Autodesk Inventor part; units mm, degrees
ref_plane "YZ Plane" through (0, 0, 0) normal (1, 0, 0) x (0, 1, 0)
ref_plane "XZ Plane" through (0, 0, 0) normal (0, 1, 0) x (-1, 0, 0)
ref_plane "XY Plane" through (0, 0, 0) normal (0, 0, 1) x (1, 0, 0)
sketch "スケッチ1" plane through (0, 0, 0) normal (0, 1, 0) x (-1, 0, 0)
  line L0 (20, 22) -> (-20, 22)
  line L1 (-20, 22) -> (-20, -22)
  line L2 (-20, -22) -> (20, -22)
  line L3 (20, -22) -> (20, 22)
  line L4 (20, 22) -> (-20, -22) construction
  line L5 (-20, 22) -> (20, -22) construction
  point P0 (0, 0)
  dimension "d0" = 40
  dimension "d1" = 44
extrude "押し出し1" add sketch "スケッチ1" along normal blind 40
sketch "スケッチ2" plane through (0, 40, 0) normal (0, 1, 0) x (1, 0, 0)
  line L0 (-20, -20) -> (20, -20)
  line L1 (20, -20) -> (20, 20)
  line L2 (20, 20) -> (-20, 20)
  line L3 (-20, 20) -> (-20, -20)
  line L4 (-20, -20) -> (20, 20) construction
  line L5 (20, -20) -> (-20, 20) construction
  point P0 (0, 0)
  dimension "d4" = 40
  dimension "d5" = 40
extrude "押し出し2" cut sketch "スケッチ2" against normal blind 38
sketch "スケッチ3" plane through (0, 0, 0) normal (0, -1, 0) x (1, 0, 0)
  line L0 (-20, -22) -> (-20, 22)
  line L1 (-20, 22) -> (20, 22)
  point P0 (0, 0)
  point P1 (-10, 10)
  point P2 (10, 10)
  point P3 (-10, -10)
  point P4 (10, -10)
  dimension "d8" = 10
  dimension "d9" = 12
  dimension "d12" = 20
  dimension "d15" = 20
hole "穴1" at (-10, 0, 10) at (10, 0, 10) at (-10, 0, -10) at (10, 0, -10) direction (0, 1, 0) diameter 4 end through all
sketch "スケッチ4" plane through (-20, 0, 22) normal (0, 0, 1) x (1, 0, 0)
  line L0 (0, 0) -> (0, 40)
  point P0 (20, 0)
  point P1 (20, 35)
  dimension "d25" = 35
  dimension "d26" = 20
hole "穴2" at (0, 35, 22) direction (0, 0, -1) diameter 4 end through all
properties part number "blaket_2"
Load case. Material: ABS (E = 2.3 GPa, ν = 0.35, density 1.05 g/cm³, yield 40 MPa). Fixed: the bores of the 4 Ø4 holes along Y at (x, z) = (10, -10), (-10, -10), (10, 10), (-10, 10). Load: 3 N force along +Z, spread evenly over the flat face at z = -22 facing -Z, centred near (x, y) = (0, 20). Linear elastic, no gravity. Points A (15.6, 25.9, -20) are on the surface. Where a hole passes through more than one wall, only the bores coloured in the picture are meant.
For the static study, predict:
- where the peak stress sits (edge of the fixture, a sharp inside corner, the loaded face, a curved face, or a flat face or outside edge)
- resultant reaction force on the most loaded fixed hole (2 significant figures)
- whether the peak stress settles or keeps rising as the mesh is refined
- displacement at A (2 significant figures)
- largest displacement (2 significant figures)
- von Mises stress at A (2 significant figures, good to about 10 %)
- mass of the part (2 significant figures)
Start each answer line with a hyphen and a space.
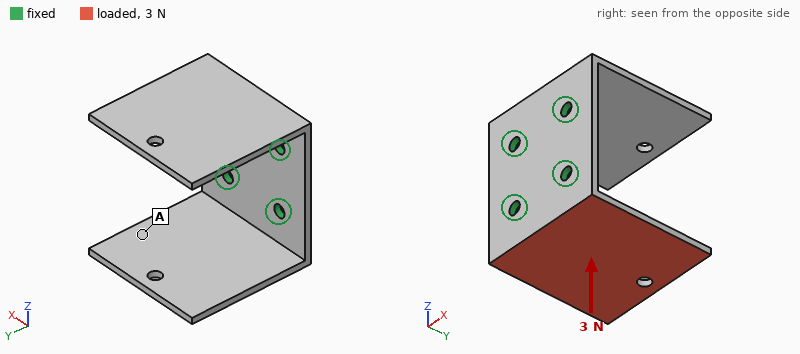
- edge of the fixture
- 1.4 N
- keeps rising
- 0.37 mm
- 0.65 mm
- 0.29 MPa
- 9.9 g
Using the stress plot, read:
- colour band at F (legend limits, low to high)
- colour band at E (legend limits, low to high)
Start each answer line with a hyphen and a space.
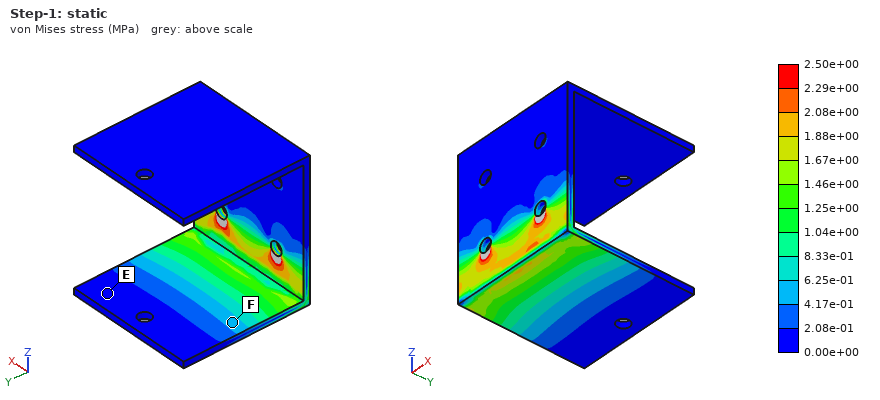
- 4.17e-01 to 6.25e-01 MPa
- 0.00e+00 to 2.08e-01 MPa
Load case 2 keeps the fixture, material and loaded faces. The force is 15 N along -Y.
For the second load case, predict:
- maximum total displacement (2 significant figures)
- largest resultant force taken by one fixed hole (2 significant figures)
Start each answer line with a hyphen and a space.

- 0.70 mm
- 8.2 N
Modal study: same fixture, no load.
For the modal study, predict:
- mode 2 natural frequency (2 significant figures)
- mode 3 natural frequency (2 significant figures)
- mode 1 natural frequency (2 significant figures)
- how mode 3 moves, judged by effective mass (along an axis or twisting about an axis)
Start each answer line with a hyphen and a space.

- 230 Hz
- 580 Hz
- 230 Hz
- along X
